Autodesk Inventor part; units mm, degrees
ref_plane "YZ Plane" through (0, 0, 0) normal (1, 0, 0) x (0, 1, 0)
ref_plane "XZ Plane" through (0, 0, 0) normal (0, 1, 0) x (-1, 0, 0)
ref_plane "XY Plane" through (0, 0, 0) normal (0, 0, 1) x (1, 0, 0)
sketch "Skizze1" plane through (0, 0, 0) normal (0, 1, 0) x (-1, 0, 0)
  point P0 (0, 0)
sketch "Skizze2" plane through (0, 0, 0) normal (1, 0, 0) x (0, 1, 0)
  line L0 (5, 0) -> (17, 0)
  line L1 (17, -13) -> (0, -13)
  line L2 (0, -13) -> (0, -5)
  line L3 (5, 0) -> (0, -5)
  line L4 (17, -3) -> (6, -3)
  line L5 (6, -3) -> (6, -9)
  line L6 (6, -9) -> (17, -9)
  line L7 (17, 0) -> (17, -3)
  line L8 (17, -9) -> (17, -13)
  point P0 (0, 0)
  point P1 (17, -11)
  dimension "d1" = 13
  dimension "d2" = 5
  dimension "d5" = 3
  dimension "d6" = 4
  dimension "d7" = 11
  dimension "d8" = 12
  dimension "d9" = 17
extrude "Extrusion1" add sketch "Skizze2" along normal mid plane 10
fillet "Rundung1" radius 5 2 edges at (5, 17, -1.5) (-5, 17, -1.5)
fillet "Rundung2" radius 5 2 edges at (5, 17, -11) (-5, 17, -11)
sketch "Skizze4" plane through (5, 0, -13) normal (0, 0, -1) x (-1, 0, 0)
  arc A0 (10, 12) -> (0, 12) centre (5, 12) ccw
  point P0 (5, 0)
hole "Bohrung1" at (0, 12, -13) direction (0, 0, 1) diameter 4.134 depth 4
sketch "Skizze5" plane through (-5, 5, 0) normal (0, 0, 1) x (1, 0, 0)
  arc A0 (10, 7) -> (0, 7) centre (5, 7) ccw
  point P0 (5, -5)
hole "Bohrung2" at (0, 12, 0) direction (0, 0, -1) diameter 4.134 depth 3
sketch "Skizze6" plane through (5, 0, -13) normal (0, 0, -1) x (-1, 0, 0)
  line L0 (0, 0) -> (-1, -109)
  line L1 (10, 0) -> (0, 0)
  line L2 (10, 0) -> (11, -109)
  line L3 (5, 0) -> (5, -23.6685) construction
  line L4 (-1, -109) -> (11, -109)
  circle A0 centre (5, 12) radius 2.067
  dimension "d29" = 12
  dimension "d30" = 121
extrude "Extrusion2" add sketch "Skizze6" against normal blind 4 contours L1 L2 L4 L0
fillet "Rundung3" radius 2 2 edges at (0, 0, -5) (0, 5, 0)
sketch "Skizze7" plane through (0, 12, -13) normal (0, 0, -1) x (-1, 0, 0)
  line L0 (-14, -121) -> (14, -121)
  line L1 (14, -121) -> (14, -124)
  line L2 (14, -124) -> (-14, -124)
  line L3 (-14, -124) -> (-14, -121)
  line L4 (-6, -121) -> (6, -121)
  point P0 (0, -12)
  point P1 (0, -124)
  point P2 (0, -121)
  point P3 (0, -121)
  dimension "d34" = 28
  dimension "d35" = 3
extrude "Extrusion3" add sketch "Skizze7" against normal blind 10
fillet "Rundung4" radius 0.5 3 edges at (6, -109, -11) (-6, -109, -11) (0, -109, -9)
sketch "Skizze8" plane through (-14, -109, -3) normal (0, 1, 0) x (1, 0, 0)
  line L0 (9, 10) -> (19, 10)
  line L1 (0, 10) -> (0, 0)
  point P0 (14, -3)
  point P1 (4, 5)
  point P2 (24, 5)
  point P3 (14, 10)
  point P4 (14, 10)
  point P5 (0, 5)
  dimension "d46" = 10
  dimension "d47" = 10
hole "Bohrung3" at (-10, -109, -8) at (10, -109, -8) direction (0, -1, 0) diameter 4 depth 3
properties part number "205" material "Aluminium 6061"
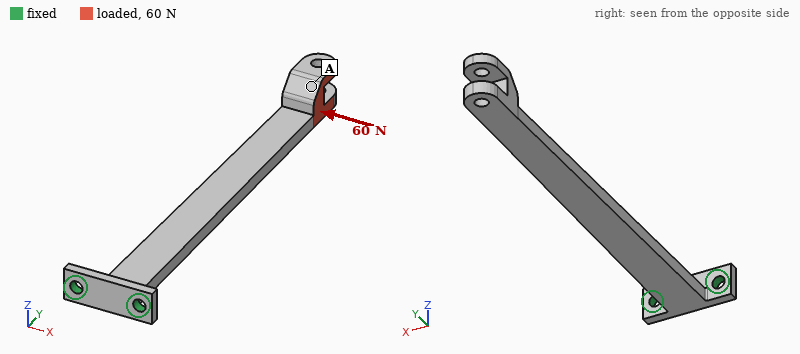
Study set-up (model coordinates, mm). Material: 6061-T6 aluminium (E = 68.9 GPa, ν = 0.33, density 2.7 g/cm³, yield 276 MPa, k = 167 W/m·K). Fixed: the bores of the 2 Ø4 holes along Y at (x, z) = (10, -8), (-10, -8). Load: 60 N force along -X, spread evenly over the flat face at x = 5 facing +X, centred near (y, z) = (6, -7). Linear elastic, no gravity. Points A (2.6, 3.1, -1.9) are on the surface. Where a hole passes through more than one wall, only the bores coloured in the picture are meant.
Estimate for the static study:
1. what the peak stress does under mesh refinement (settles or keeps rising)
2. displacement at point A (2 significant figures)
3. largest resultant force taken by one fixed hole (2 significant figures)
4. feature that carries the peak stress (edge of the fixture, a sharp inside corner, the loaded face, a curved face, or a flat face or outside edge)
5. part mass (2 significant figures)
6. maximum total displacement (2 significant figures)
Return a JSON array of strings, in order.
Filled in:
["keeps rising", "1.1 mm", "480 N", "a sharp inside corner", "18 g", "1.3 mm"]
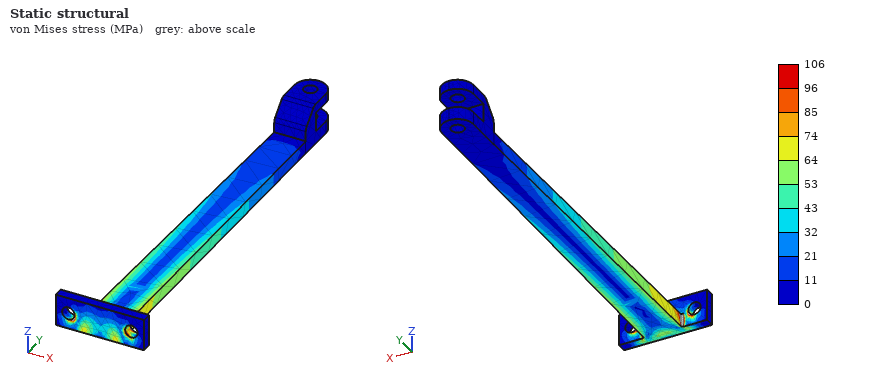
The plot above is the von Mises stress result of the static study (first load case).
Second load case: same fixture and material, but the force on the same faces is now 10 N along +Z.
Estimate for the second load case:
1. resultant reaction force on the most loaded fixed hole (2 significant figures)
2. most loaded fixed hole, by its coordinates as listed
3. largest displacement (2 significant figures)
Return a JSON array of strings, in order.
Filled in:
["15 N", "(10, -8)", "1.6 mm"]
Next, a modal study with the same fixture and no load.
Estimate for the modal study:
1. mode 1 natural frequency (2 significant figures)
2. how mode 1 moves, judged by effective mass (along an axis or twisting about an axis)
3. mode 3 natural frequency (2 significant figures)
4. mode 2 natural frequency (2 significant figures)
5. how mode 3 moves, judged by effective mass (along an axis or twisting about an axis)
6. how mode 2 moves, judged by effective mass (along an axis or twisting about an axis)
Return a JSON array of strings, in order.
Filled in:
["170 Hz", "along Z", "1100 Hz", "490 Hz", "along Z", "along X"]
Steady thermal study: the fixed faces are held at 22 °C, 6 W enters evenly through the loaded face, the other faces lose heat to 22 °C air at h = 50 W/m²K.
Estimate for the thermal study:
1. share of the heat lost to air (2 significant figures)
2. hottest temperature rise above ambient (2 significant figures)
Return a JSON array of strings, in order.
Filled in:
["73 %", "42 K"]
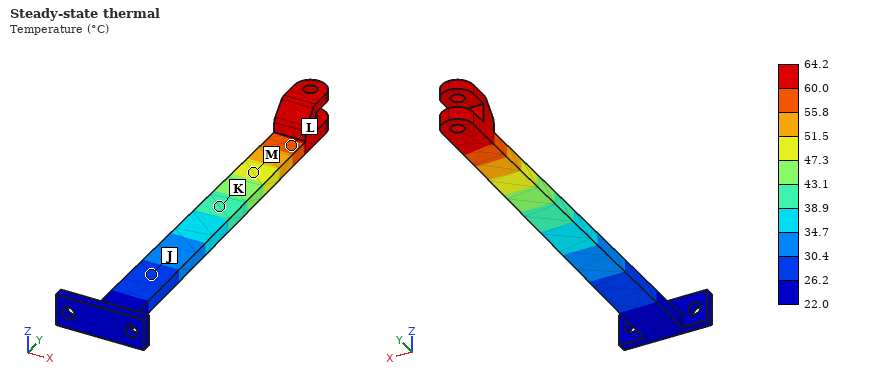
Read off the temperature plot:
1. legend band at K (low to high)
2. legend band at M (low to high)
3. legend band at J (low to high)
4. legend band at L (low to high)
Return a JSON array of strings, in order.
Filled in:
["38.9 to 43.1 °C", "47.3 to 51.5 °C", "26.2 to 30.4 °C", "55.8 to 60.0 °C"]
